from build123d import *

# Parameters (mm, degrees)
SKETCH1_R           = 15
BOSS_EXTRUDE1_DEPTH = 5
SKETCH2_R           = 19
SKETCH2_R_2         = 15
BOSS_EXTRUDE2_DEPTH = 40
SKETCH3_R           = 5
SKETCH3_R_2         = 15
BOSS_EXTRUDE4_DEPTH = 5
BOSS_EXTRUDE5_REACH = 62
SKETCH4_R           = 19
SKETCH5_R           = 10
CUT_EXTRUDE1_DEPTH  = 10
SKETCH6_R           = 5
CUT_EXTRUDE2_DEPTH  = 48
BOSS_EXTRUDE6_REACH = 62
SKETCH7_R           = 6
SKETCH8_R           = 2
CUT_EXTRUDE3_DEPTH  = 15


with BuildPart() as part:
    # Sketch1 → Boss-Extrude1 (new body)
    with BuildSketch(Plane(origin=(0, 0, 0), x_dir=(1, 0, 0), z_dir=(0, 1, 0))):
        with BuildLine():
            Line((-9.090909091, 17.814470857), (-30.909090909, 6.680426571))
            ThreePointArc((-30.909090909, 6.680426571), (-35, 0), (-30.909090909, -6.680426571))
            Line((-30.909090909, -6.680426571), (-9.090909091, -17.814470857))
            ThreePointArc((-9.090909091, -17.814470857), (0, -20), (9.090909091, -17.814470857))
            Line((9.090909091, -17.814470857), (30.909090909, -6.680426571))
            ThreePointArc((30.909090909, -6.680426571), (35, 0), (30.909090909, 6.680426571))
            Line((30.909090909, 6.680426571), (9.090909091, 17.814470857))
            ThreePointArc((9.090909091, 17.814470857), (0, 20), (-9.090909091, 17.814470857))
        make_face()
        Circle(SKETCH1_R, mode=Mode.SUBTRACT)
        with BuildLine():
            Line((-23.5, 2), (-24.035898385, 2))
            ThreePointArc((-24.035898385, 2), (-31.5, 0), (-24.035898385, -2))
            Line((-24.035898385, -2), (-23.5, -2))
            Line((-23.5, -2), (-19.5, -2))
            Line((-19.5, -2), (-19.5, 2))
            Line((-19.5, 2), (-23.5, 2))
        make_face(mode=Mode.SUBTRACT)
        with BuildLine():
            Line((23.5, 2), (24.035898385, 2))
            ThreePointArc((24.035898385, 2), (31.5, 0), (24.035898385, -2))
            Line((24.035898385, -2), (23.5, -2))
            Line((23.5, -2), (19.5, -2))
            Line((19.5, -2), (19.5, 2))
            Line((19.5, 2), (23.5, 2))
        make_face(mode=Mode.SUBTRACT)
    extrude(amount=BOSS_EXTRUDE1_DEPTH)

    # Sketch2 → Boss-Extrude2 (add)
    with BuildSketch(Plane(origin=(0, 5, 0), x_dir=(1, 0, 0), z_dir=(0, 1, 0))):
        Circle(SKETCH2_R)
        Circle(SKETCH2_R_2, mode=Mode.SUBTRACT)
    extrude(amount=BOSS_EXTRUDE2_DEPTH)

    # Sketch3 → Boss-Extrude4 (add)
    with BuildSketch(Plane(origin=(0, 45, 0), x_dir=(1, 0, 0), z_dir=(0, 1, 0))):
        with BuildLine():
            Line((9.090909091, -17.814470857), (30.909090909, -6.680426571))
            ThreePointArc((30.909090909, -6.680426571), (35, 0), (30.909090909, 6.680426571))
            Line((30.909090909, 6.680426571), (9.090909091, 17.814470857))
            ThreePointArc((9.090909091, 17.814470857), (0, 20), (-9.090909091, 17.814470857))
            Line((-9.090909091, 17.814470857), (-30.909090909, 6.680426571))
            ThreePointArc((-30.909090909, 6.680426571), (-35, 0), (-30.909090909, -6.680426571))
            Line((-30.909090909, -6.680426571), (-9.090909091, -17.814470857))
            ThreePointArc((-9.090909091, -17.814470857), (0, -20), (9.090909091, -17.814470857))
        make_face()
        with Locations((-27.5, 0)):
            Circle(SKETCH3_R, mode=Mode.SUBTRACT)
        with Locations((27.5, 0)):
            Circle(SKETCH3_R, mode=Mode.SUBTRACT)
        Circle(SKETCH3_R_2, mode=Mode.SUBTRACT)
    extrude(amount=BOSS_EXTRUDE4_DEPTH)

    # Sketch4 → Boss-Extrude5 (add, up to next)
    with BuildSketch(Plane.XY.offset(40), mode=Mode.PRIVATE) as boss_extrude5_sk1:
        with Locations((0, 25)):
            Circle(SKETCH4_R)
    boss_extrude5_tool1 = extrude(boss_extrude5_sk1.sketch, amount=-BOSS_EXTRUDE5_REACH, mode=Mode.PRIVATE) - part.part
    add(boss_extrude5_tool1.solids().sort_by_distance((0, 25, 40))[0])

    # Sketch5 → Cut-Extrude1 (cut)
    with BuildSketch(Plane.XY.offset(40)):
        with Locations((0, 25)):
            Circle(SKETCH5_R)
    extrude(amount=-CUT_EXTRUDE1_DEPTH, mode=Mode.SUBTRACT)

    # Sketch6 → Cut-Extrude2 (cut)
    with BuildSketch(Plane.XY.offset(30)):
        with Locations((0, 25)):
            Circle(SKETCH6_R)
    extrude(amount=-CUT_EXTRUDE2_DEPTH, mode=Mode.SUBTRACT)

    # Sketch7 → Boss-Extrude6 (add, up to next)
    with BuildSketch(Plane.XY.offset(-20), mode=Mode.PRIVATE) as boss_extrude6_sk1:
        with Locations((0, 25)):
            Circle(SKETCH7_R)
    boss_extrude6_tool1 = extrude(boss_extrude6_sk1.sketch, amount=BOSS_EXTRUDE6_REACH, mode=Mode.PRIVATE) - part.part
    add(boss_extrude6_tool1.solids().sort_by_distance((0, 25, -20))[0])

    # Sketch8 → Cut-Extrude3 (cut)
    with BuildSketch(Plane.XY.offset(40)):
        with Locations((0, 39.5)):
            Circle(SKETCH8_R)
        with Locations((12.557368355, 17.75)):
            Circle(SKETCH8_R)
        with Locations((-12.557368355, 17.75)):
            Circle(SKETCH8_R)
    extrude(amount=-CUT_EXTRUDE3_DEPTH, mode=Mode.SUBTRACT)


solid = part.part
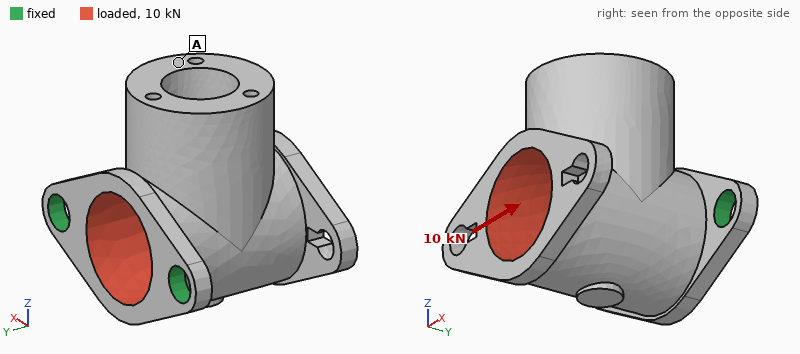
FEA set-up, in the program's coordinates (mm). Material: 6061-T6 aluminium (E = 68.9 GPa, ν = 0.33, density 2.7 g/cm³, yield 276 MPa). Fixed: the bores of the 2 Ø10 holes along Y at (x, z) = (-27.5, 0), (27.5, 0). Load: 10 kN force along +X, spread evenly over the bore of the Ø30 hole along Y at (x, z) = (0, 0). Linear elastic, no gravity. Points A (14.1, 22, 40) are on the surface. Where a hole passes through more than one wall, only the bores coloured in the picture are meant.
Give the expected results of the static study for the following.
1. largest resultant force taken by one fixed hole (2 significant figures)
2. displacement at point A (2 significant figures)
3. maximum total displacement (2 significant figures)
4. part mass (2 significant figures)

7.4 kN
0.085 mm
0.17 mm
130 g
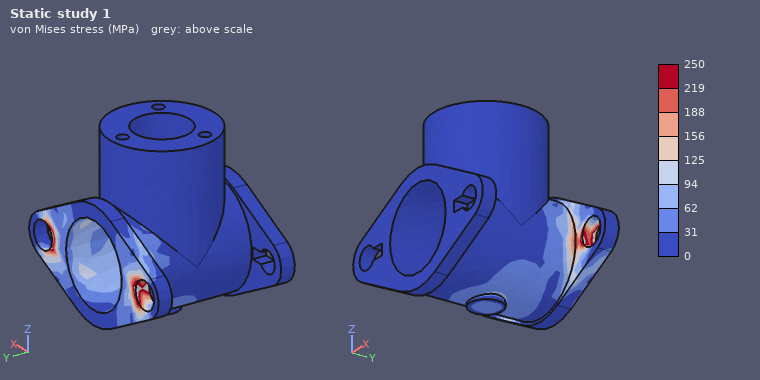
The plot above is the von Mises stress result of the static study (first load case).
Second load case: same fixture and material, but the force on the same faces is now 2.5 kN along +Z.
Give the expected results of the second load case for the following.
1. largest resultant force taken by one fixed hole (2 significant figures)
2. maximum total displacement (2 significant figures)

1.3 kN
0.41 mm
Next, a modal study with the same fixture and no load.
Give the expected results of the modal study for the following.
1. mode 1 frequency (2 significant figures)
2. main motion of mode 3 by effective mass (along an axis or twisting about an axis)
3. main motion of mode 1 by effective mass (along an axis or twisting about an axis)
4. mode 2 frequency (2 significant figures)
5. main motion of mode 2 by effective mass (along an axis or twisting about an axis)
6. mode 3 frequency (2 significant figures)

1200 Hz
along Y
along Z
3900 Hz
along X
6400 Hz
